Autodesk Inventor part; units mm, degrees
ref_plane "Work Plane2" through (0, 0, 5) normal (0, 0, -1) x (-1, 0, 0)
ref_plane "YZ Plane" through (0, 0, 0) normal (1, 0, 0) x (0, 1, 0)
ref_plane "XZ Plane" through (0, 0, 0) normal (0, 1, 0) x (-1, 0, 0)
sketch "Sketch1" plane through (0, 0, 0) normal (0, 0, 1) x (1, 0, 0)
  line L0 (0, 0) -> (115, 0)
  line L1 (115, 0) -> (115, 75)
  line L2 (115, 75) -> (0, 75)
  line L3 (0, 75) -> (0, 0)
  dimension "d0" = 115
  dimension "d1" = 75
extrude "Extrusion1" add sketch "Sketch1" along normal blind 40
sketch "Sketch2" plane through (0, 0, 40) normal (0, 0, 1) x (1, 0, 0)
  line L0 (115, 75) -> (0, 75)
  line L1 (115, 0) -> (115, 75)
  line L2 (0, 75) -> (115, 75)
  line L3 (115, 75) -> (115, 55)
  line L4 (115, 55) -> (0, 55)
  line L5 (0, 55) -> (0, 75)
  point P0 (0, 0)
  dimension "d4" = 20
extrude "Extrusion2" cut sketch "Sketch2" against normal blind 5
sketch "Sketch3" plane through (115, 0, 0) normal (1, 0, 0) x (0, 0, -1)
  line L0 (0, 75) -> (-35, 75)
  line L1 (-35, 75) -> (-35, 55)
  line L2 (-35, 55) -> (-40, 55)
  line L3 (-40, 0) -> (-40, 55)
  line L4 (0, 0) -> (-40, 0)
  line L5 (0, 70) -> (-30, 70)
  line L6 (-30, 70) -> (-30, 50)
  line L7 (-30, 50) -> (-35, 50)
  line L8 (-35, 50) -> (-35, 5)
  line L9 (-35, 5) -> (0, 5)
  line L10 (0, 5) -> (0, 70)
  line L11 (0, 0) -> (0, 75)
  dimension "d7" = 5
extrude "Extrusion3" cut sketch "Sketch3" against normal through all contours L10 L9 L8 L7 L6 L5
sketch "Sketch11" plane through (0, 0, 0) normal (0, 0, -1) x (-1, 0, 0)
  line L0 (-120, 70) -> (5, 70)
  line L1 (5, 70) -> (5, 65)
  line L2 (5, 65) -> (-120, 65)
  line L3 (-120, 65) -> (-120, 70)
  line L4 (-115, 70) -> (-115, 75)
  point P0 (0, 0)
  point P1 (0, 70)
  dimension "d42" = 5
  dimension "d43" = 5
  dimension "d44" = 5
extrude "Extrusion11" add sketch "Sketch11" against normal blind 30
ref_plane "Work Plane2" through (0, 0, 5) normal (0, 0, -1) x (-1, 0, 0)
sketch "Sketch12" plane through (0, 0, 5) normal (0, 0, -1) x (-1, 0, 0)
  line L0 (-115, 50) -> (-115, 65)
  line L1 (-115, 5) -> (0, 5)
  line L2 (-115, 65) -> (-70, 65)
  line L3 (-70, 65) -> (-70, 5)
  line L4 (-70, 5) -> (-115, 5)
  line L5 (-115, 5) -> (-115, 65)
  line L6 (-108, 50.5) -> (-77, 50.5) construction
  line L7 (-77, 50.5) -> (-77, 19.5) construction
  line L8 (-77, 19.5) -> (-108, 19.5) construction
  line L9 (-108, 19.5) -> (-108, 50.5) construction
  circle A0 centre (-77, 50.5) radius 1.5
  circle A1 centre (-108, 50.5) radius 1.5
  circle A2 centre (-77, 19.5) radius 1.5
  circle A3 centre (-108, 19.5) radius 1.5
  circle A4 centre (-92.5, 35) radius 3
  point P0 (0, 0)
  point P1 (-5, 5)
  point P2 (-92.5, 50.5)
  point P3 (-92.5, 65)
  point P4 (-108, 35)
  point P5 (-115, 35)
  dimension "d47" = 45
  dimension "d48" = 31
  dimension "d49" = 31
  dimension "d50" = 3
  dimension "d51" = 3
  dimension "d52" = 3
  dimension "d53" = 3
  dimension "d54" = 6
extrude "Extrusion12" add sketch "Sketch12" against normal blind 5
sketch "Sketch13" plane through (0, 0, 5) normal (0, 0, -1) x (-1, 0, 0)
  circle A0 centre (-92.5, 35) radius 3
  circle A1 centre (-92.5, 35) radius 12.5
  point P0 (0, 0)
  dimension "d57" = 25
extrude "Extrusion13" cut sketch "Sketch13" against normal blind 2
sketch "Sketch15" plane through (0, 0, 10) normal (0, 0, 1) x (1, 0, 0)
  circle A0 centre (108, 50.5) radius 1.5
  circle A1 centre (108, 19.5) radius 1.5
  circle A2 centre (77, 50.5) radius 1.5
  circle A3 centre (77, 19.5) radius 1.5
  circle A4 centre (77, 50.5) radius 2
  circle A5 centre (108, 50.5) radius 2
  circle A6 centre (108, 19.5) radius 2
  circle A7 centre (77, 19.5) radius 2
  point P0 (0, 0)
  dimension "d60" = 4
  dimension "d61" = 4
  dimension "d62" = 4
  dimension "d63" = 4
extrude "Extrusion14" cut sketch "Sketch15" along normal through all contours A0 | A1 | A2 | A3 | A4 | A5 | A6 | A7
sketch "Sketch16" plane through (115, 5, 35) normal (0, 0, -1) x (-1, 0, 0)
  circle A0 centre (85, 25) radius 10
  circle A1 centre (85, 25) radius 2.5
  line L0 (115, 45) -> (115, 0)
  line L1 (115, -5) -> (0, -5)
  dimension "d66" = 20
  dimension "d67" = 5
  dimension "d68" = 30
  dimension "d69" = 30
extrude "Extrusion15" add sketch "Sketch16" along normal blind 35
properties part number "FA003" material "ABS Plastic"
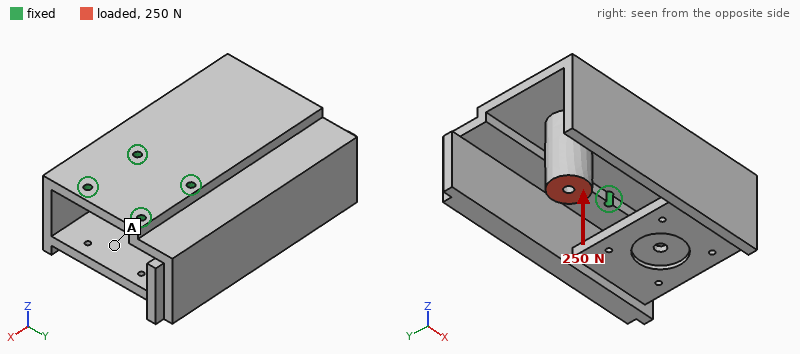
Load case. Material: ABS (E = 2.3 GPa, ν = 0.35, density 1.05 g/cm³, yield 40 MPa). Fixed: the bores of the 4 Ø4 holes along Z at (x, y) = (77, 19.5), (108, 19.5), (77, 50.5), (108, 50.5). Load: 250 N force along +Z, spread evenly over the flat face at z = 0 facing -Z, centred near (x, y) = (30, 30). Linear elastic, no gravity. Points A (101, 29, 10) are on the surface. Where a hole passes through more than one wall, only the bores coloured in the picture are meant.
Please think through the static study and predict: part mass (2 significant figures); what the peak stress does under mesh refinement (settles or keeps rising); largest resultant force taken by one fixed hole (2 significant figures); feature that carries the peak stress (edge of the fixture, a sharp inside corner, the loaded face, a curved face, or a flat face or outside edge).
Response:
130 g
keeps rising
270 N
edge of the fixture
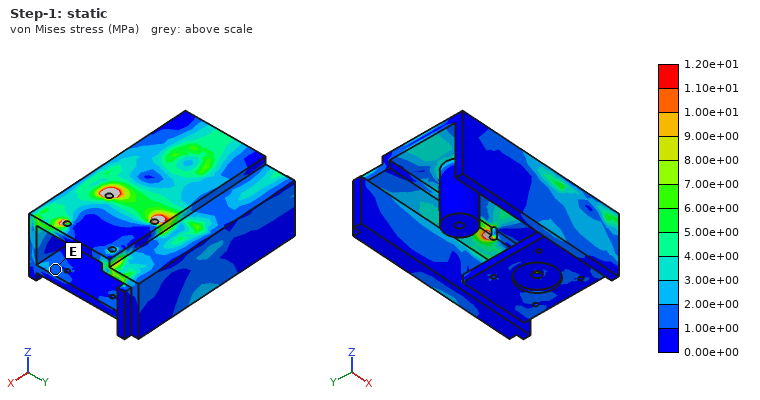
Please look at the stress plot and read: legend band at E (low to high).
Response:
1.00e+00 to 2.00e+00 MPa
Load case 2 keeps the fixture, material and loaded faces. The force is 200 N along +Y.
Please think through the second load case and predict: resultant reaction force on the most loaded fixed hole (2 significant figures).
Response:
320 N
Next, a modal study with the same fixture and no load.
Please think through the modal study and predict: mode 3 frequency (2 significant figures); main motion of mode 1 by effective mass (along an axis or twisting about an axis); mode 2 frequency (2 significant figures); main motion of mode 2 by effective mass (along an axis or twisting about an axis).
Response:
640 Hz
along Z
370 Hz
along Y
